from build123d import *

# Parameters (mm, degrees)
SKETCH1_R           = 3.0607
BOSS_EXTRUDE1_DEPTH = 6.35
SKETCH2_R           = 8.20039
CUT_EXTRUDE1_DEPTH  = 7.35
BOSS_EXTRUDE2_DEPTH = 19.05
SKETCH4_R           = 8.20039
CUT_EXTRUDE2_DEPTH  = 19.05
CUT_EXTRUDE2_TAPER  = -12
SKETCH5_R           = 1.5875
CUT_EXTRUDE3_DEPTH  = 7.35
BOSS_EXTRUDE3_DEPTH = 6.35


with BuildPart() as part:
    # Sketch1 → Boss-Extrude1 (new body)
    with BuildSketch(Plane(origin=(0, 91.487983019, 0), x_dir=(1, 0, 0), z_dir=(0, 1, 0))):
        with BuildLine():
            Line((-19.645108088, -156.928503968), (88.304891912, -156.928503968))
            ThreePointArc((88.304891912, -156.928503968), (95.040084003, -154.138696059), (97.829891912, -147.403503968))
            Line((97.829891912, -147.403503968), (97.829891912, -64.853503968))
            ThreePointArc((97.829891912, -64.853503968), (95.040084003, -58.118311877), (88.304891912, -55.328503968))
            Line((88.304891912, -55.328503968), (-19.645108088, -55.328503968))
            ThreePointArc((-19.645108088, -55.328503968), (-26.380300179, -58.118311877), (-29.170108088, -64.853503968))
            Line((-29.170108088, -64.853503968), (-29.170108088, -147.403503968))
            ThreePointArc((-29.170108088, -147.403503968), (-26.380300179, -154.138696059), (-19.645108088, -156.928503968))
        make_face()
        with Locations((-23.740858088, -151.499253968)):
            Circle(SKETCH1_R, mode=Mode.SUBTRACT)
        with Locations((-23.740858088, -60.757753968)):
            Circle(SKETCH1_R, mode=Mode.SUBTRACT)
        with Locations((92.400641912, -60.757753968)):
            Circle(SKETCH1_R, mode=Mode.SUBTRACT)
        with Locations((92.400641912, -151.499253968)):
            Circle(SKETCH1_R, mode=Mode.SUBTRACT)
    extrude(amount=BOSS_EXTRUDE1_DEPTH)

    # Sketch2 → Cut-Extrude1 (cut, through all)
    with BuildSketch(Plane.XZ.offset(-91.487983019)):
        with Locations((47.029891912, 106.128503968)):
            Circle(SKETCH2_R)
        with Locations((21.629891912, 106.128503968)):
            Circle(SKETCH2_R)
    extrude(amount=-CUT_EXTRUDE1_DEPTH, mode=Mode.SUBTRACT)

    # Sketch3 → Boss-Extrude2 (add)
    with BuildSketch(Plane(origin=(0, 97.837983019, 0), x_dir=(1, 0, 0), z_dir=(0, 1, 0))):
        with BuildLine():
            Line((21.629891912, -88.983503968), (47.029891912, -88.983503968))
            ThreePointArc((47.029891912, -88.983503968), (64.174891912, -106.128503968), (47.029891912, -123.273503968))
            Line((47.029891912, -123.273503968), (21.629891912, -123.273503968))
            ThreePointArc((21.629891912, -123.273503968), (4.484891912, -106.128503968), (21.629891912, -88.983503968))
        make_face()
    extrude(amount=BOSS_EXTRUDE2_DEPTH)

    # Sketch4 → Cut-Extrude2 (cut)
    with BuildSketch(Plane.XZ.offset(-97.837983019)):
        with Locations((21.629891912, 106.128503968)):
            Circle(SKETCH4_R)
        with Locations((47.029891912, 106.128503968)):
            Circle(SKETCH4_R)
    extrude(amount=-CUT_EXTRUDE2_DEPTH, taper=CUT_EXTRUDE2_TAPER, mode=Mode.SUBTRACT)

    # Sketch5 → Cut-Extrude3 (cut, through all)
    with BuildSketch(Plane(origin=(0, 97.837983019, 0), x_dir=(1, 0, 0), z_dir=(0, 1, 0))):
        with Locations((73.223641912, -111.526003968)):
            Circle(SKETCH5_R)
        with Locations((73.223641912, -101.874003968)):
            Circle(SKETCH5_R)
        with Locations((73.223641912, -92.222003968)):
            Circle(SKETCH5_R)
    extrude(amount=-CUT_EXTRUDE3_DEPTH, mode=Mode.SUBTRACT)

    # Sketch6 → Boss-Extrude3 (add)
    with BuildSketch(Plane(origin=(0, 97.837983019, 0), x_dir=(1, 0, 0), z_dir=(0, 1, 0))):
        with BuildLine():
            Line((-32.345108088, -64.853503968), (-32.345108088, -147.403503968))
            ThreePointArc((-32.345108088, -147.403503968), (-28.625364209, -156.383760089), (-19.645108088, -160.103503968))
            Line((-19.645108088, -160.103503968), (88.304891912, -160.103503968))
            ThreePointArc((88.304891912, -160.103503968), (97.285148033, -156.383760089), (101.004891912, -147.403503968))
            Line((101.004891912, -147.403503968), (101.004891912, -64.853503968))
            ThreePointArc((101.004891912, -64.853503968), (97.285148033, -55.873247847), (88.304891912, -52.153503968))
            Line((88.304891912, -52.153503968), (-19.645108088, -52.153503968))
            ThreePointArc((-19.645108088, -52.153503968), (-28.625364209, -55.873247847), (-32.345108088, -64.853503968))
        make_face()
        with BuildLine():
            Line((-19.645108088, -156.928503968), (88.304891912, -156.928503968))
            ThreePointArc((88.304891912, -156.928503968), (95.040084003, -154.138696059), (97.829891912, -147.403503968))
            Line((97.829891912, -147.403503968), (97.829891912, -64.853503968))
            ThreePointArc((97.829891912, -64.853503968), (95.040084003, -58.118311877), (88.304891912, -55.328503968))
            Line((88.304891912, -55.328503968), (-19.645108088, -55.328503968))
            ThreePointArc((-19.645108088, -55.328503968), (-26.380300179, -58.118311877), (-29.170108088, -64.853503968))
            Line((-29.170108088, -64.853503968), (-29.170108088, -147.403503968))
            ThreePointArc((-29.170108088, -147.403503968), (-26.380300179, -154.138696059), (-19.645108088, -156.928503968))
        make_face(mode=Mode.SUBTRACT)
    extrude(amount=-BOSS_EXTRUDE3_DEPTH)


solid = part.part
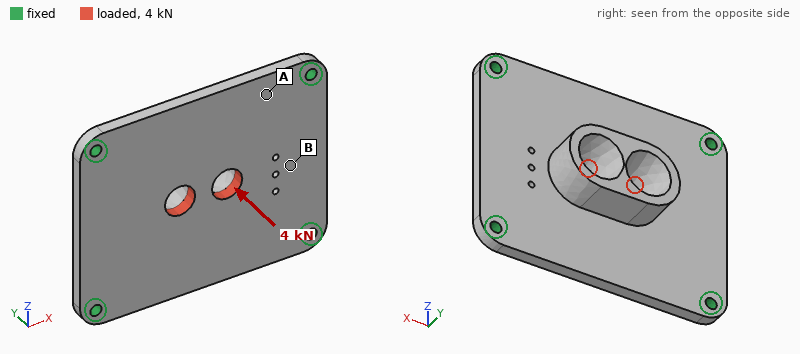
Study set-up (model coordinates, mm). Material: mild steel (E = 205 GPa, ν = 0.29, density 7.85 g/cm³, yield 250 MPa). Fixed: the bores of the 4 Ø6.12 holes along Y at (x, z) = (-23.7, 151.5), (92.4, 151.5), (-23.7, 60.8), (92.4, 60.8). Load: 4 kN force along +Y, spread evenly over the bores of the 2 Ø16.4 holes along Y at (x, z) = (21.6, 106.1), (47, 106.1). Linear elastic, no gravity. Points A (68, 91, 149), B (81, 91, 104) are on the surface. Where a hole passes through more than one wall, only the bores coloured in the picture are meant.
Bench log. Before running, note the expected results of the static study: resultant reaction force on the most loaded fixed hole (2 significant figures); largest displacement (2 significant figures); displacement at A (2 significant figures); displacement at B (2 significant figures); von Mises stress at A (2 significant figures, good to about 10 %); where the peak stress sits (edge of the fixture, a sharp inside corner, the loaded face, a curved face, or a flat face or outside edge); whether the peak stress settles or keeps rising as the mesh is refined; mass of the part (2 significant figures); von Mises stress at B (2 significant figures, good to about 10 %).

1.1 kN
69 µm
25 µm
43 µm
13 MPa
edge of the fixture
keeps rising
850 g
37 MPa
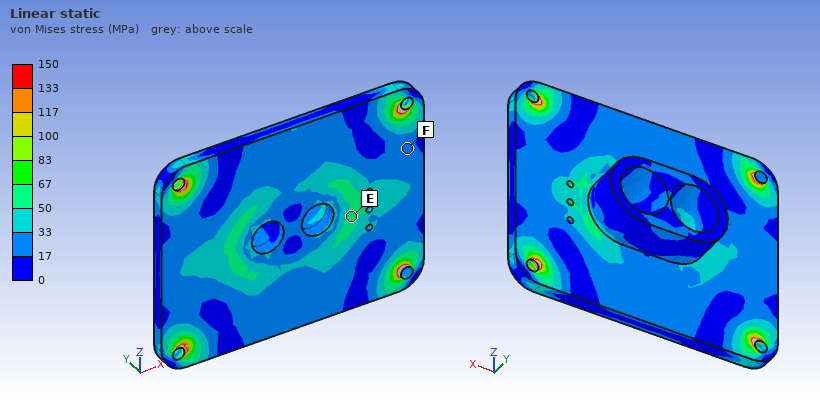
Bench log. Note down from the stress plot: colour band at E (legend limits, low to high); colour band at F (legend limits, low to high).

50 to 67 MPa
17 to 33 MPa
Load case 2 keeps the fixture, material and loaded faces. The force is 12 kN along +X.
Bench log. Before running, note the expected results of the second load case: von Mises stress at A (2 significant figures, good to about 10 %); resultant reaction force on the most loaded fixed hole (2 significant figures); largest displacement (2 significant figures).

13 MPa
3.3 kN
8.7 µm
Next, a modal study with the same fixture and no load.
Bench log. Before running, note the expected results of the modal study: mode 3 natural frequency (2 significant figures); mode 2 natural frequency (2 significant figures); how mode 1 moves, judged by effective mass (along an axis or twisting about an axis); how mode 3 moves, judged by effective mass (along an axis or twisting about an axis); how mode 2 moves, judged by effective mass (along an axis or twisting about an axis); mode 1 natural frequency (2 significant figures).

3600 Hz
2800 Hz
along Y
twisting about Z
twisting about X
1800 Hz
